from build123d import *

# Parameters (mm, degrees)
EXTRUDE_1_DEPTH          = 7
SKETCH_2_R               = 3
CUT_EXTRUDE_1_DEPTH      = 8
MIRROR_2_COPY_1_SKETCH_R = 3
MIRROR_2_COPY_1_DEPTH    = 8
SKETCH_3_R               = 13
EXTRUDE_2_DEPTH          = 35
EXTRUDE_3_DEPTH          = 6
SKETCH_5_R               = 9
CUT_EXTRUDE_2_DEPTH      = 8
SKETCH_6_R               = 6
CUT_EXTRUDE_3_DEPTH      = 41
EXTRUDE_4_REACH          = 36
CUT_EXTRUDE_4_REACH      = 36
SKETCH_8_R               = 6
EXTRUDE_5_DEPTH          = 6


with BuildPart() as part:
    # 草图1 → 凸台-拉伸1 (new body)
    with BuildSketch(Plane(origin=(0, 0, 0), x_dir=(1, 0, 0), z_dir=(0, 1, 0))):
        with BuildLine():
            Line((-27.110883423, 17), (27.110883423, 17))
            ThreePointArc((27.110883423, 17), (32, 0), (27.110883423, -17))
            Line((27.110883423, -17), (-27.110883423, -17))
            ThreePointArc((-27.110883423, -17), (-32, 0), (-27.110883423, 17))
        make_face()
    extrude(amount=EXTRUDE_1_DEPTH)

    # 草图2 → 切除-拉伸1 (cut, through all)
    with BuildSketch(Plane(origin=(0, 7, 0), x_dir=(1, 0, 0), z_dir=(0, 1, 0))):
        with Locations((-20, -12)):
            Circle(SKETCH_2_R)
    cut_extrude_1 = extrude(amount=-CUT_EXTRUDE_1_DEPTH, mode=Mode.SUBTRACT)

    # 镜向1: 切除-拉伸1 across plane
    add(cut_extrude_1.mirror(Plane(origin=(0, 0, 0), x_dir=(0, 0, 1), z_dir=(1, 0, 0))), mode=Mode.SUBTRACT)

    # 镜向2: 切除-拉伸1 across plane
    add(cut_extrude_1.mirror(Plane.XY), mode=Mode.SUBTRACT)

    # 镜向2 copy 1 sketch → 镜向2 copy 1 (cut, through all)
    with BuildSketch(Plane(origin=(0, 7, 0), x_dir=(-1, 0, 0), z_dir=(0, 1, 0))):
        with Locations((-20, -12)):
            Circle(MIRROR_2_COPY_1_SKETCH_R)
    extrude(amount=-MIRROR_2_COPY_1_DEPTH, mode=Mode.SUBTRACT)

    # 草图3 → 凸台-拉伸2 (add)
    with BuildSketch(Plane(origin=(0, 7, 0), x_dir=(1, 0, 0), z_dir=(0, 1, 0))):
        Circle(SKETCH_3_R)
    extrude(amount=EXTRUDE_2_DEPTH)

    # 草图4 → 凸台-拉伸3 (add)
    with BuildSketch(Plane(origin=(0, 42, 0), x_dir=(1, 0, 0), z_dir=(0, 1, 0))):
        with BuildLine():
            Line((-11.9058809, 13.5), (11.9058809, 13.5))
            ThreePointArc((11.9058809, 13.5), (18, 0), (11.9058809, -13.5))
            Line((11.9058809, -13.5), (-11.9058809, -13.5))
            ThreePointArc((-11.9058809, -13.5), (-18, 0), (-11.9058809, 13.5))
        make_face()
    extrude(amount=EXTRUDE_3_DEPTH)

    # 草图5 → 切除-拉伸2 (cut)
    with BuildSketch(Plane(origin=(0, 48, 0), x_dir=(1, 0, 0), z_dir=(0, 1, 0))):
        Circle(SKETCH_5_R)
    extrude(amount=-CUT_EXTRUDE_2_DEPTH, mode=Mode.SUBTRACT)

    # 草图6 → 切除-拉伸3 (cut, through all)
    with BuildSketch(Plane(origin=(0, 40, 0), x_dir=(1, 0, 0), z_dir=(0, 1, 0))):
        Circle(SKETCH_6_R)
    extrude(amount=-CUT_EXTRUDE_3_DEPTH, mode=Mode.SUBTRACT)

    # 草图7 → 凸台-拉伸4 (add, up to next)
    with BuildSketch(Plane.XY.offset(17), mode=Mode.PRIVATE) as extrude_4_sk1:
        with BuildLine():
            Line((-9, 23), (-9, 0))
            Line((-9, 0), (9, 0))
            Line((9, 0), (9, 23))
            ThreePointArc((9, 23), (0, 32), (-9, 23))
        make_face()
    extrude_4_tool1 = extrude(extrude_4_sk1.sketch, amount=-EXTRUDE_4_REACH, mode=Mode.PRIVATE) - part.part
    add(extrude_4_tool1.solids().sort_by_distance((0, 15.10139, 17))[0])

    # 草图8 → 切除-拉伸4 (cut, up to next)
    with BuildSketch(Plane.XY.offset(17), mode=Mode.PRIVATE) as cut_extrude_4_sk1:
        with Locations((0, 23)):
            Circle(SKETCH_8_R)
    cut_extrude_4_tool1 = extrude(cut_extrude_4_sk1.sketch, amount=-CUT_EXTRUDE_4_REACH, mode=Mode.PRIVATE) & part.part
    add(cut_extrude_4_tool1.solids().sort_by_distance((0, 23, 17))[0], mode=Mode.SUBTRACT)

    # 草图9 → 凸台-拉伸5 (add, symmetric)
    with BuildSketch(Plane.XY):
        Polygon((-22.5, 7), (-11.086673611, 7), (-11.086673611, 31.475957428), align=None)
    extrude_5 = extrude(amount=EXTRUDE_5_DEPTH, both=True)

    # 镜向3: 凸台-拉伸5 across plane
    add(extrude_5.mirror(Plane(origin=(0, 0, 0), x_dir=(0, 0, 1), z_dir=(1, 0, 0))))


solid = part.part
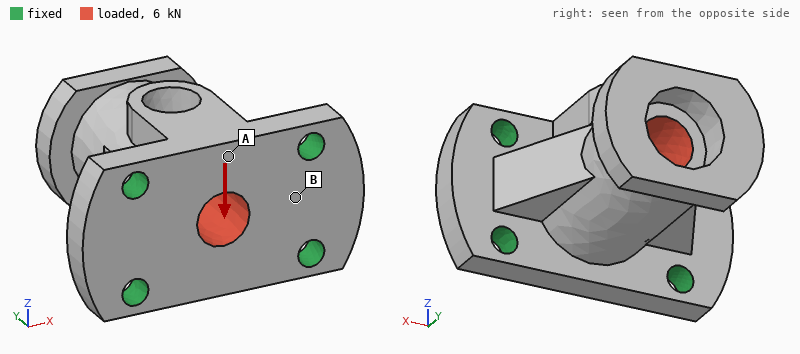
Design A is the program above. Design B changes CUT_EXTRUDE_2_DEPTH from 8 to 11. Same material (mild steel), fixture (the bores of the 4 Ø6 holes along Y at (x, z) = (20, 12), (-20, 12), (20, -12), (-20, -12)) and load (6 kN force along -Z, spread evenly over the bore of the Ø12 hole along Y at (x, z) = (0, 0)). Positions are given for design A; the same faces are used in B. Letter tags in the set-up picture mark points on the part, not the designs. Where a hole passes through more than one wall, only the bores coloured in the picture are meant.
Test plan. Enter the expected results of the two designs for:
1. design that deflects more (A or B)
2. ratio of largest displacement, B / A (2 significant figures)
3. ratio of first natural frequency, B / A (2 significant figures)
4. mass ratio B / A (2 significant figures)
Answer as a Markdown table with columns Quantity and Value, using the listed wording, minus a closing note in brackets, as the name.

| Quantity | Value |
|---|---|
| design that deflects more | A |
| ratio of largest displacement, B / A | 0.87 |
| ratio of first natural frequency, B / A | 1.0 |
| mass ratio B / A | 0.99 |
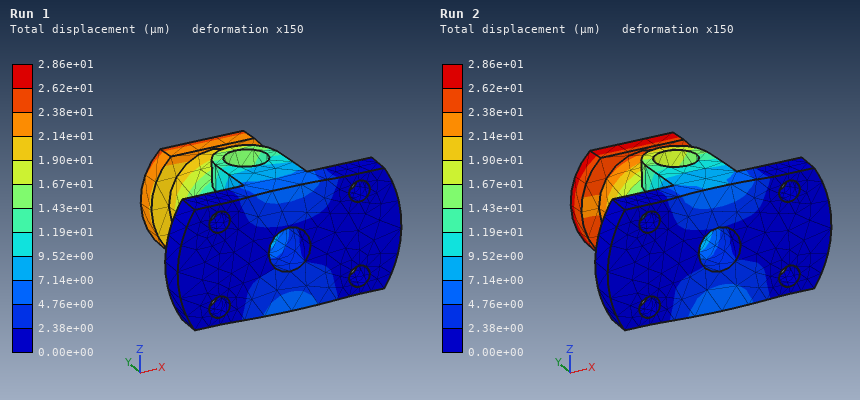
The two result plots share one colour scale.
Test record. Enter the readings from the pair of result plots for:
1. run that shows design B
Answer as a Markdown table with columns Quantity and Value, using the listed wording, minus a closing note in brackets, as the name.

| Quantity | Value |
|---|---|
| run that shows design B | Run 1 |
